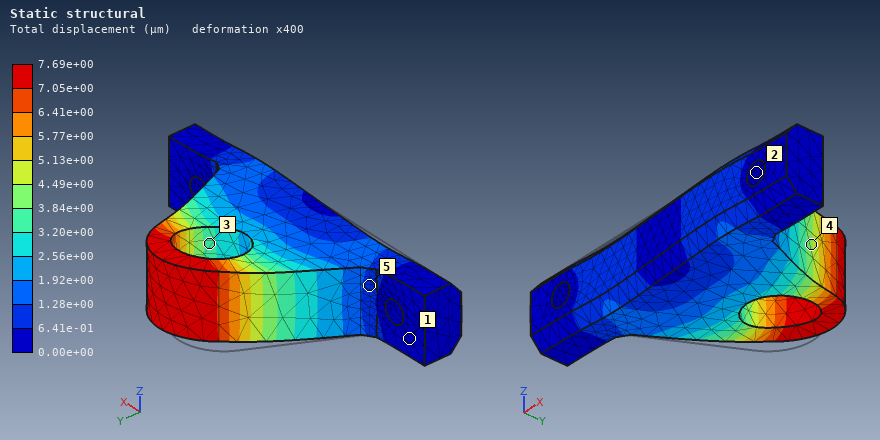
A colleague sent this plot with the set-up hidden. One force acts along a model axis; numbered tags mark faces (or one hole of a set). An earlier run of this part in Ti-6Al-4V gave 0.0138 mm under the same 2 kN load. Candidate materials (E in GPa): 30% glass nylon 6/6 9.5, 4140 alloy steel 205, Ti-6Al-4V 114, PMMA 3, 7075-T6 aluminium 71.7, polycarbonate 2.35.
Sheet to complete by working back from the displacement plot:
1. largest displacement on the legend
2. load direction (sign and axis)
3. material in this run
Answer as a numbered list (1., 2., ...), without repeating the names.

1. 7.69e+00 µm
2. +X
3. 4140 alloy steel
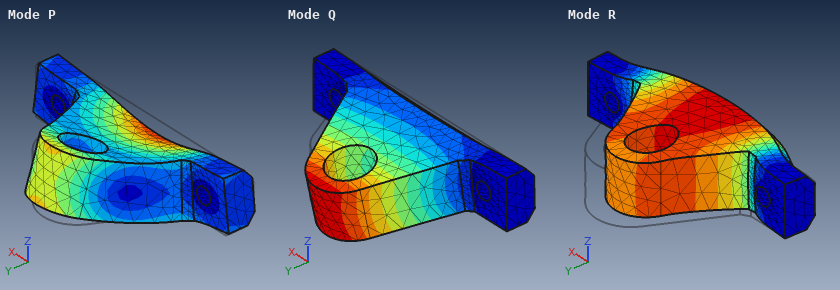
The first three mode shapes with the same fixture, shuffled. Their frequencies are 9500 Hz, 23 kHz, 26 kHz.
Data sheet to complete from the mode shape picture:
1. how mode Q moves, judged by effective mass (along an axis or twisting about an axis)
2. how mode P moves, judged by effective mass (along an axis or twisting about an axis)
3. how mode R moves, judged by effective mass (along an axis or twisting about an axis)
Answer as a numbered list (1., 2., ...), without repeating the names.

1. along Z
2. along Z
3. along Y
